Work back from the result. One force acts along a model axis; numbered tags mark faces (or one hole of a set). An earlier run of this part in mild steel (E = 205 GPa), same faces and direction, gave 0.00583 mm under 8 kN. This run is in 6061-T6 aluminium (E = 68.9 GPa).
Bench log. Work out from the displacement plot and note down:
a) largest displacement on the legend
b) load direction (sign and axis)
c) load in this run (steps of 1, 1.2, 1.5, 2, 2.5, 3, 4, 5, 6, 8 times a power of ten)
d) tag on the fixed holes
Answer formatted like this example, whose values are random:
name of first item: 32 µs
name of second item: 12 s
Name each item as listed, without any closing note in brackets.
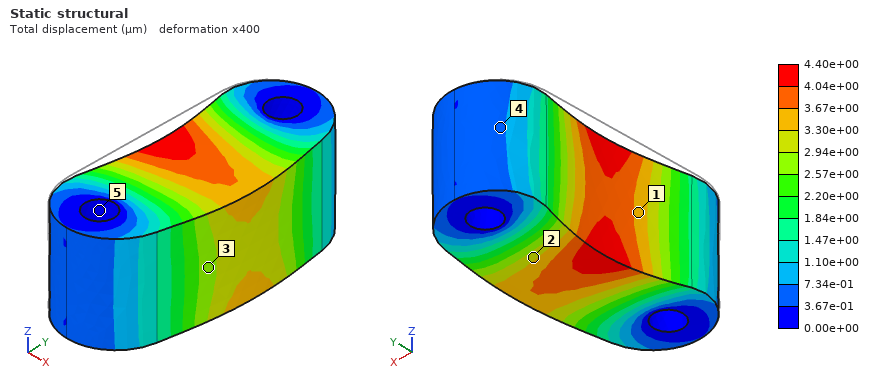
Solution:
largest displacement on the legend: 4.40e+00 µm
load direction: +X
load in this run: 2 kN
tag on the fixed holes: 5
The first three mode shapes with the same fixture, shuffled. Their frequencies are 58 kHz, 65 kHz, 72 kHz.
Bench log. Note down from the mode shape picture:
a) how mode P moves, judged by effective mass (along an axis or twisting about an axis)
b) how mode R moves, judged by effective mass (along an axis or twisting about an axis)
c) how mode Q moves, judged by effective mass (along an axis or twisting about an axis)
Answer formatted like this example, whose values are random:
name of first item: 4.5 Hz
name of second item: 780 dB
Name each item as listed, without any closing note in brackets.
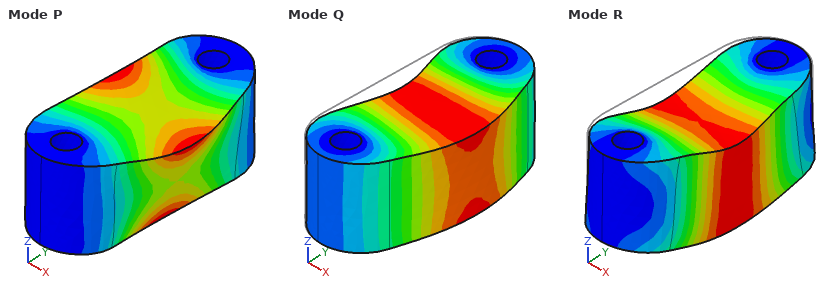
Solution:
how mode P moves, judged by effective mass: twisting about Y
how mode R moves, judged by effective mass: along Z
how mode Q moves, judged by effective mass: along X
